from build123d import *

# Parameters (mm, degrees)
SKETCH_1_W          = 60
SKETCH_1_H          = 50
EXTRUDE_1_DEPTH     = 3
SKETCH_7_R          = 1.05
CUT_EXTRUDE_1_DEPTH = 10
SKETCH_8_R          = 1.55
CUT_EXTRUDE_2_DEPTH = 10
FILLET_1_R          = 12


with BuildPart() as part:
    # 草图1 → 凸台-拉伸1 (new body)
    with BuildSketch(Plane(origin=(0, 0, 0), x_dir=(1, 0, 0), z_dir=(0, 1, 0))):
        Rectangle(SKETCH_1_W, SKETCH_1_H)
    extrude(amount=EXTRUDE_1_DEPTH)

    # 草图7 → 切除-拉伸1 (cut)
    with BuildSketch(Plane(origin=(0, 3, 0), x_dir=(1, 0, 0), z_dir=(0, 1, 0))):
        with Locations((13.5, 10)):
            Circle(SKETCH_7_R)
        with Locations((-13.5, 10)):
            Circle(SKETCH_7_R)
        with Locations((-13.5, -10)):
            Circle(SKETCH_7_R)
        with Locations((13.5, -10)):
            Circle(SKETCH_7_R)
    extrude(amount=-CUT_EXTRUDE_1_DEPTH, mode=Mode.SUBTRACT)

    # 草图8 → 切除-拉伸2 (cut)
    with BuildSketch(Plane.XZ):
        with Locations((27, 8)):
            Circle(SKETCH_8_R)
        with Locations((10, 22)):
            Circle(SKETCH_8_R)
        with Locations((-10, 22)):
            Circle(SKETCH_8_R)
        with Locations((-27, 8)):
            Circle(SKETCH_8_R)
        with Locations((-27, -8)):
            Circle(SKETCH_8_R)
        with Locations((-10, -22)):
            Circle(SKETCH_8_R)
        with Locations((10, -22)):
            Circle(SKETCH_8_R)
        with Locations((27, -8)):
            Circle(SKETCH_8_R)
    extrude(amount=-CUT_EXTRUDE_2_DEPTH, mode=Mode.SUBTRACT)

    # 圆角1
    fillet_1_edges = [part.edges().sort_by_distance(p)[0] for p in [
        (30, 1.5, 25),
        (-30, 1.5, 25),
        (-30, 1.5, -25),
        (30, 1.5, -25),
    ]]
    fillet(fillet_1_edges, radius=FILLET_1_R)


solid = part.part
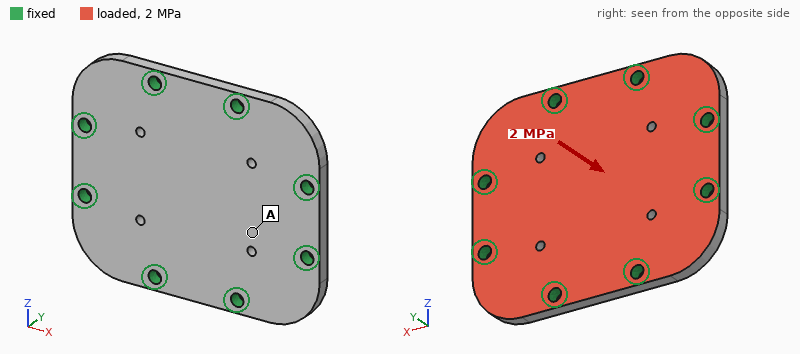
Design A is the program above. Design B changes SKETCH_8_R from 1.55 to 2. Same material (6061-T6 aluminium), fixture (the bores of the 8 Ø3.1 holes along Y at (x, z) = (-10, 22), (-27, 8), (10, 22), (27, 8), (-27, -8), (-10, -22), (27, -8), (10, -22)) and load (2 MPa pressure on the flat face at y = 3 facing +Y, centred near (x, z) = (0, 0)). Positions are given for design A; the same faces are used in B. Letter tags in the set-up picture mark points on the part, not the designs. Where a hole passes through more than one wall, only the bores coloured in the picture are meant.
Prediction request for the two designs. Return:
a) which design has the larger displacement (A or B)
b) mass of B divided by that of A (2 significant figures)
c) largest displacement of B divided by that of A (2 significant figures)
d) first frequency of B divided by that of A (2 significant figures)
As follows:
A
0.99
0.89
1.1
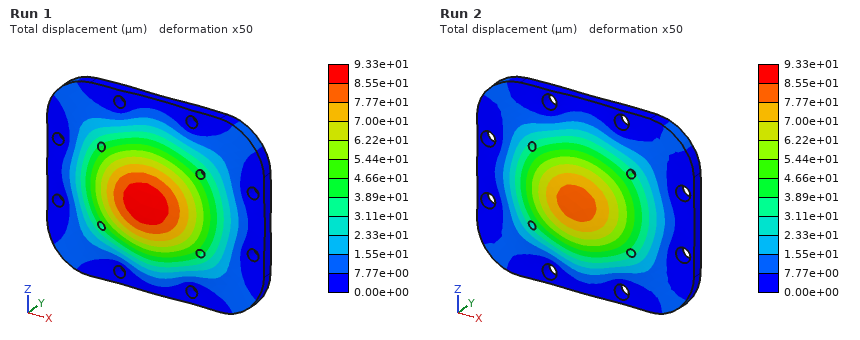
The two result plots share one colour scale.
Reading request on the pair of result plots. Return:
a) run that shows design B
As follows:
Run 2
